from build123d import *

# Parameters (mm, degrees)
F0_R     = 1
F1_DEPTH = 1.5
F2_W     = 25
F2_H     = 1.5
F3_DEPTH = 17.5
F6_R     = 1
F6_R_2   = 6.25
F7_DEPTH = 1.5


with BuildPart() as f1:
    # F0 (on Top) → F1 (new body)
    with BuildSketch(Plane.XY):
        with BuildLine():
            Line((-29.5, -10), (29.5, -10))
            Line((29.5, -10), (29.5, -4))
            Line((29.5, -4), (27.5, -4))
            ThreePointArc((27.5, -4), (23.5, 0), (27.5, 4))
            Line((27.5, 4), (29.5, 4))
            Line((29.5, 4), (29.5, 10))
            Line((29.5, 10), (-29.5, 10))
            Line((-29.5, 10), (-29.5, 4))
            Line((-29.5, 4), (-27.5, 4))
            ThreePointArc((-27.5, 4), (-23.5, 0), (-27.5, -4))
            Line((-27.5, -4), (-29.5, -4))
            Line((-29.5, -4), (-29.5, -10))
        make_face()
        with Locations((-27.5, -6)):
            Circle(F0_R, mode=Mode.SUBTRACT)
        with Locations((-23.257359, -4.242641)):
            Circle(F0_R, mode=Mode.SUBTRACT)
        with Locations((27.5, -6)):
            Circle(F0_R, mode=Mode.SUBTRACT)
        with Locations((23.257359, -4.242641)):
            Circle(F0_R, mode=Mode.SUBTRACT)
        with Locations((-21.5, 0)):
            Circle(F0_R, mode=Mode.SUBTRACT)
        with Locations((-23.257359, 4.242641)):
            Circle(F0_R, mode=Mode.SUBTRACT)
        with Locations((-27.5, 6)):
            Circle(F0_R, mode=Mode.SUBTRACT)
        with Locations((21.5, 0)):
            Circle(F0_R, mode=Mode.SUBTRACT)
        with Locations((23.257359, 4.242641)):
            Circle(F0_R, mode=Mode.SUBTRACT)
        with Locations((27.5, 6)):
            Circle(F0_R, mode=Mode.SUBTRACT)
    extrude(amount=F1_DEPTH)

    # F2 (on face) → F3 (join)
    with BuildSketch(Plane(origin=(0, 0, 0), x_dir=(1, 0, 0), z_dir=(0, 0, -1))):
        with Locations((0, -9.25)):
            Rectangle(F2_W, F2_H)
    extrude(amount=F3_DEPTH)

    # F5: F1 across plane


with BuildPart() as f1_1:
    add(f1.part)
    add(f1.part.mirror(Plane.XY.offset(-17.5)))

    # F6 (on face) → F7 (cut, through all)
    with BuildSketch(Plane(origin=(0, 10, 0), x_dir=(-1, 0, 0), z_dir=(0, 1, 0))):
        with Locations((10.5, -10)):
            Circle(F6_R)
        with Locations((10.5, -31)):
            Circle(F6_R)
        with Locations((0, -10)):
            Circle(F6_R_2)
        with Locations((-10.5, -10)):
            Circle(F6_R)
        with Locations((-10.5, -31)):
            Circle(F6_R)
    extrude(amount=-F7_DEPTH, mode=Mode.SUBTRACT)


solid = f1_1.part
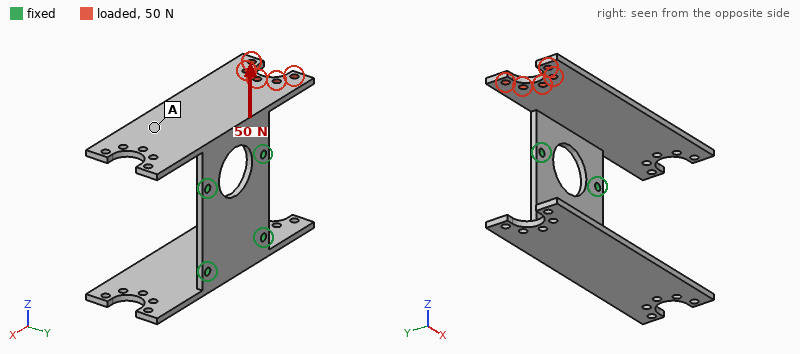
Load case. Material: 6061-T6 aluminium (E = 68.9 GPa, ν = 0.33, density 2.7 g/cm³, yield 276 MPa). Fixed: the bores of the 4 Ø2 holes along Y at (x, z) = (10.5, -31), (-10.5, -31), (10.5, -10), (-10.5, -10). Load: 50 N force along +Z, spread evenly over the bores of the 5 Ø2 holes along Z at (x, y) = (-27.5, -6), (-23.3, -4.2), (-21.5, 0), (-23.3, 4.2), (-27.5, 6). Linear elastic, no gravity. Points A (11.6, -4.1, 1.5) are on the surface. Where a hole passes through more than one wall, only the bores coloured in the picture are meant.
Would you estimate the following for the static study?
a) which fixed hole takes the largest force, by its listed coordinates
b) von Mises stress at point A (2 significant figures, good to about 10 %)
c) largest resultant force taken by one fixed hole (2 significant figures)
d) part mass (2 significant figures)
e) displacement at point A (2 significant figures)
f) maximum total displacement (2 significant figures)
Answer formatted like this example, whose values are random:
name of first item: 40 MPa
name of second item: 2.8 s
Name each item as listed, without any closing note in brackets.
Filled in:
which fixed hole takes the largest force, by its listed coordinates: (-10.5, -10)
von Mises stress at point A: 15 MPa
largest resultant force taken by one fixed hole: 82 N
part mass: 12 g
displacement at point A: 0.17 mm
maximum total displacement: 0.86 mm
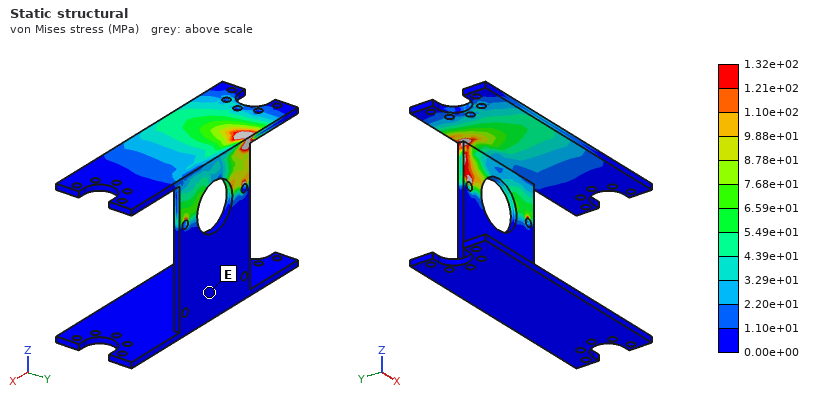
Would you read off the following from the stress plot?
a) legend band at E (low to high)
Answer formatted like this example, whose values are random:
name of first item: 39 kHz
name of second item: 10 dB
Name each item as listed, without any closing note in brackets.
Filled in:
legend band at E: 0.00e+00 to 1.10e+01 MPa
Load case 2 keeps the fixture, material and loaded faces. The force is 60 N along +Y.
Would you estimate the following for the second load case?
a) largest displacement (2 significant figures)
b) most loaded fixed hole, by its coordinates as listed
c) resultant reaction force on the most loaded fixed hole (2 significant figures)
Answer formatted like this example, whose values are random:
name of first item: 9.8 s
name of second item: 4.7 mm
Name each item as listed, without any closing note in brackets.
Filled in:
largest displacement: 0.47 mm
most loaded fixed hole, by its coordinates as listed: (-10.5, -10)
resultant reaction force on the most loaded fixed hole: 99 N
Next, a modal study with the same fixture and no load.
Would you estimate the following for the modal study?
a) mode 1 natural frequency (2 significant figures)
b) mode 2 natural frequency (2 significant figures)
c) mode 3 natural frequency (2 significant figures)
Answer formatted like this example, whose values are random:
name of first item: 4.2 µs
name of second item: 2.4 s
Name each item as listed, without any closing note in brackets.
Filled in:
mode 1 natural frequency: 1000 Hz
mode 2 natural frequency: 1600 Hz
mode 3 natural frequency: 1600 Hz
